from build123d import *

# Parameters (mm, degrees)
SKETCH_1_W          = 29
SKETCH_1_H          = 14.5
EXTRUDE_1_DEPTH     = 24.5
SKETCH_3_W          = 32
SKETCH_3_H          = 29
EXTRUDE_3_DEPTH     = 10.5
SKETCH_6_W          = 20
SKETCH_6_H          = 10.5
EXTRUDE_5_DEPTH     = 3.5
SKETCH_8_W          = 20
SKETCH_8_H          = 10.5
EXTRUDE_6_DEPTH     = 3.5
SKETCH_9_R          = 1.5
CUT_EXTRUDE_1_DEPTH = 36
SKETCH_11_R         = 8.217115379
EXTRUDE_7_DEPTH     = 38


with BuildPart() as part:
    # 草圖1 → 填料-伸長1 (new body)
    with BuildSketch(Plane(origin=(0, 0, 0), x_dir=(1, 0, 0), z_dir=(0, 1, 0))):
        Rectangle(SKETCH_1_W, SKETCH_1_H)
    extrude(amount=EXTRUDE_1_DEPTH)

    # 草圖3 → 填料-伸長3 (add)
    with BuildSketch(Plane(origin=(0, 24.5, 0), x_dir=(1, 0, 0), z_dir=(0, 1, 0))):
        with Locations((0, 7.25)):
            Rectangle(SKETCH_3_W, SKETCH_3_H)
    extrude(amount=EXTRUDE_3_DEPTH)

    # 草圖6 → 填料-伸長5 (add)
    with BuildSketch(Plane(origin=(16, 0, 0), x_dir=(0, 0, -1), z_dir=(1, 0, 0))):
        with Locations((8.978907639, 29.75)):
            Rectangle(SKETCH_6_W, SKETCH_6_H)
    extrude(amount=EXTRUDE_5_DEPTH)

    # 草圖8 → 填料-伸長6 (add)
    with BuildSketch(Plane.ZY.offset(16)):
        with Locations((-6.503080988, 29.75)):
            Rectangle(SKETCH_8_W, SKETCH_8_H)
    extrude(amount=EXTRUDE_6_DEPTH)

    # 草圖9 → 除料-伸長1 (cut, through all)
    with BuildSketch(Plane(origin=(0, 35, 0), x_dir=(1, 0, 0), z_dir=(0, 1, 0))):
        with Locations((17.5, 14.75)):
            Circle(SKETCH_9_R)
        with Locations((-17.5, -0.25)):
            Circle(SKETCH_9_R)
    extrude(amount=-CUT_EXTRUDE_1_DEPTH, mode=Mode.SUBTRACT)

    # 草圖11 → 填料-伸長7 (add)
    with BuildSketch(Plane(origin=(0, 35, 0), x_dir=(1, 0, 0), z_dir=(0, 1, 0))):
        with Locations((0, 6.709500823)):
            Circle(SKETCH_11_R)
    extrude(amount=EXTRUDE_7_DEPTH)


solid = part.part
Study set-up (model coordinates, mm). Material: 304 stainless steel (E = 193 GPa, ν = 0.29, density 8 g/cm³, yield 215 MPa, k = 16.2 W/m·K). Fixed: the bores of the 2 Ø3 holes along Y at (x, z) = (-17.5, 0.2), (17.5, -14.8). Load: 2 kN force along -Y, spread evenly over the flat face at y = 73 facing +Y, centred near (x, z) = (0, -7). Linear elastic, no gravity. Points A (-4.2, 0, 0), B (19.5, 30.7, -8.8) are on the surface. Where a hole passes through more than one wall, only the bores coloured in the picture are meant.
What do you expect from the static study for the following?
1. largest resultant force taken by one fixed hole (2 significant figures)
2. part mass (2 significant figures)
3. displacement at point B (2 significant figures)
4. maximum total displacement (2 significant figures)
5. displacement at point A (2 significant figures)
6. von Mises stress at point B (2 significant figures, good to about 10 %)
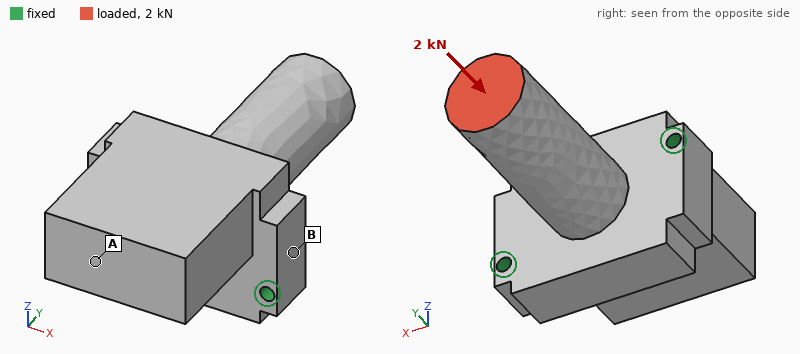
1.0 kN
240 g
0.68 µm
3.9 µm
1.7 µm
14 MPa
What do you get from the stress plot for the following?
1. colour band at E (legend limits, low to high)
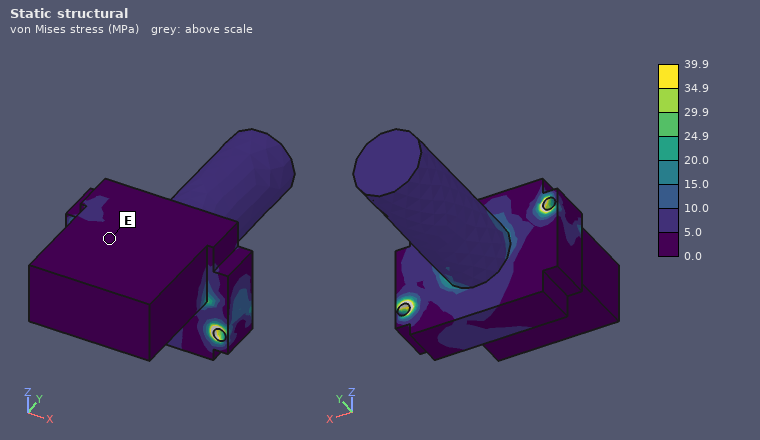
0.0 to 5.0 MPa
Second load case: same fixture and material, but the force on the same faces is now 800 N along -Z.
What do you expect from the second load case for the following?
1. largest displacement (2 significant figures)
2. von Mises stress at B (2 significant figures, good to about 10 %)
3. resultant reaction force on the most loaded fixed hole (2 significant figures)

55 µm
34 MPa
590 N
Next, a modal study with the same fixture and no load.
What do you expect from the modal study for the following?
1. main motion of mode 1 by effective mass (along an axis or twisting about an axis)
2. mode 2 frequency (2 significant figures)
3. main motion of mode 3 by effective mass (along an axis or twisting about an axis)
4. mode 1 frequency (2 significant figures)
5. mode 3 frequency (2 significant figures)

twisting about X
5700 Hz
along Z
3600 Hz
7600 Hz
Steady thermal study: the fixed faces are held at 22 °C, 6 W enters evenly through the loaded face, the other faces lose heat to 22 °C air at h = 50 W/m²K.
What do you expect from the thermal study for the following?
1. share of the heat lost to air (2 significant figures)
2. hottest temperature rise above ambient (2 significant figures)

62 %
55 K
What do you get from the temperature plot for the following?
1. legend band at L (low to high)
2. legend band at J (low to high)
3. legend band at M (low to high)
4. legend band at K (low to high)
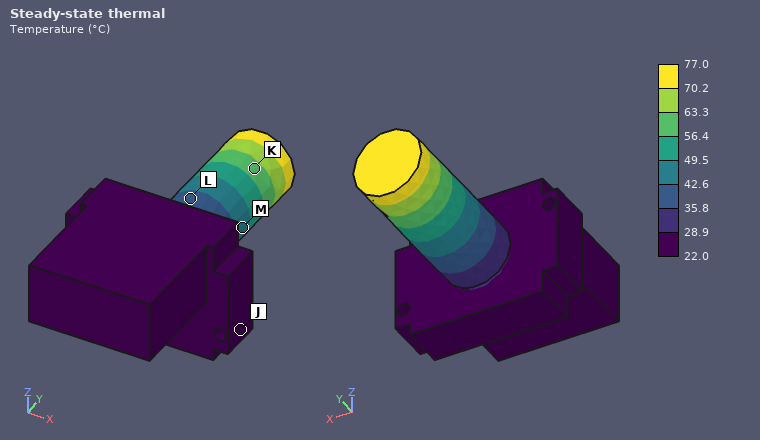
35.8 to 42.6 °C
22.0 to 28.9 °C
42.6 to 49.5 °C
56.4 to 63.3 °C
